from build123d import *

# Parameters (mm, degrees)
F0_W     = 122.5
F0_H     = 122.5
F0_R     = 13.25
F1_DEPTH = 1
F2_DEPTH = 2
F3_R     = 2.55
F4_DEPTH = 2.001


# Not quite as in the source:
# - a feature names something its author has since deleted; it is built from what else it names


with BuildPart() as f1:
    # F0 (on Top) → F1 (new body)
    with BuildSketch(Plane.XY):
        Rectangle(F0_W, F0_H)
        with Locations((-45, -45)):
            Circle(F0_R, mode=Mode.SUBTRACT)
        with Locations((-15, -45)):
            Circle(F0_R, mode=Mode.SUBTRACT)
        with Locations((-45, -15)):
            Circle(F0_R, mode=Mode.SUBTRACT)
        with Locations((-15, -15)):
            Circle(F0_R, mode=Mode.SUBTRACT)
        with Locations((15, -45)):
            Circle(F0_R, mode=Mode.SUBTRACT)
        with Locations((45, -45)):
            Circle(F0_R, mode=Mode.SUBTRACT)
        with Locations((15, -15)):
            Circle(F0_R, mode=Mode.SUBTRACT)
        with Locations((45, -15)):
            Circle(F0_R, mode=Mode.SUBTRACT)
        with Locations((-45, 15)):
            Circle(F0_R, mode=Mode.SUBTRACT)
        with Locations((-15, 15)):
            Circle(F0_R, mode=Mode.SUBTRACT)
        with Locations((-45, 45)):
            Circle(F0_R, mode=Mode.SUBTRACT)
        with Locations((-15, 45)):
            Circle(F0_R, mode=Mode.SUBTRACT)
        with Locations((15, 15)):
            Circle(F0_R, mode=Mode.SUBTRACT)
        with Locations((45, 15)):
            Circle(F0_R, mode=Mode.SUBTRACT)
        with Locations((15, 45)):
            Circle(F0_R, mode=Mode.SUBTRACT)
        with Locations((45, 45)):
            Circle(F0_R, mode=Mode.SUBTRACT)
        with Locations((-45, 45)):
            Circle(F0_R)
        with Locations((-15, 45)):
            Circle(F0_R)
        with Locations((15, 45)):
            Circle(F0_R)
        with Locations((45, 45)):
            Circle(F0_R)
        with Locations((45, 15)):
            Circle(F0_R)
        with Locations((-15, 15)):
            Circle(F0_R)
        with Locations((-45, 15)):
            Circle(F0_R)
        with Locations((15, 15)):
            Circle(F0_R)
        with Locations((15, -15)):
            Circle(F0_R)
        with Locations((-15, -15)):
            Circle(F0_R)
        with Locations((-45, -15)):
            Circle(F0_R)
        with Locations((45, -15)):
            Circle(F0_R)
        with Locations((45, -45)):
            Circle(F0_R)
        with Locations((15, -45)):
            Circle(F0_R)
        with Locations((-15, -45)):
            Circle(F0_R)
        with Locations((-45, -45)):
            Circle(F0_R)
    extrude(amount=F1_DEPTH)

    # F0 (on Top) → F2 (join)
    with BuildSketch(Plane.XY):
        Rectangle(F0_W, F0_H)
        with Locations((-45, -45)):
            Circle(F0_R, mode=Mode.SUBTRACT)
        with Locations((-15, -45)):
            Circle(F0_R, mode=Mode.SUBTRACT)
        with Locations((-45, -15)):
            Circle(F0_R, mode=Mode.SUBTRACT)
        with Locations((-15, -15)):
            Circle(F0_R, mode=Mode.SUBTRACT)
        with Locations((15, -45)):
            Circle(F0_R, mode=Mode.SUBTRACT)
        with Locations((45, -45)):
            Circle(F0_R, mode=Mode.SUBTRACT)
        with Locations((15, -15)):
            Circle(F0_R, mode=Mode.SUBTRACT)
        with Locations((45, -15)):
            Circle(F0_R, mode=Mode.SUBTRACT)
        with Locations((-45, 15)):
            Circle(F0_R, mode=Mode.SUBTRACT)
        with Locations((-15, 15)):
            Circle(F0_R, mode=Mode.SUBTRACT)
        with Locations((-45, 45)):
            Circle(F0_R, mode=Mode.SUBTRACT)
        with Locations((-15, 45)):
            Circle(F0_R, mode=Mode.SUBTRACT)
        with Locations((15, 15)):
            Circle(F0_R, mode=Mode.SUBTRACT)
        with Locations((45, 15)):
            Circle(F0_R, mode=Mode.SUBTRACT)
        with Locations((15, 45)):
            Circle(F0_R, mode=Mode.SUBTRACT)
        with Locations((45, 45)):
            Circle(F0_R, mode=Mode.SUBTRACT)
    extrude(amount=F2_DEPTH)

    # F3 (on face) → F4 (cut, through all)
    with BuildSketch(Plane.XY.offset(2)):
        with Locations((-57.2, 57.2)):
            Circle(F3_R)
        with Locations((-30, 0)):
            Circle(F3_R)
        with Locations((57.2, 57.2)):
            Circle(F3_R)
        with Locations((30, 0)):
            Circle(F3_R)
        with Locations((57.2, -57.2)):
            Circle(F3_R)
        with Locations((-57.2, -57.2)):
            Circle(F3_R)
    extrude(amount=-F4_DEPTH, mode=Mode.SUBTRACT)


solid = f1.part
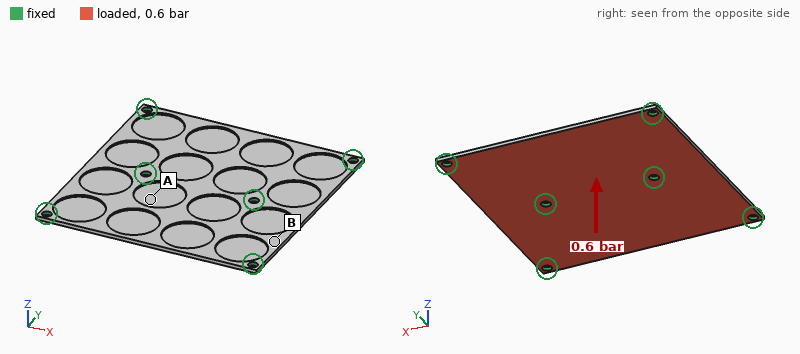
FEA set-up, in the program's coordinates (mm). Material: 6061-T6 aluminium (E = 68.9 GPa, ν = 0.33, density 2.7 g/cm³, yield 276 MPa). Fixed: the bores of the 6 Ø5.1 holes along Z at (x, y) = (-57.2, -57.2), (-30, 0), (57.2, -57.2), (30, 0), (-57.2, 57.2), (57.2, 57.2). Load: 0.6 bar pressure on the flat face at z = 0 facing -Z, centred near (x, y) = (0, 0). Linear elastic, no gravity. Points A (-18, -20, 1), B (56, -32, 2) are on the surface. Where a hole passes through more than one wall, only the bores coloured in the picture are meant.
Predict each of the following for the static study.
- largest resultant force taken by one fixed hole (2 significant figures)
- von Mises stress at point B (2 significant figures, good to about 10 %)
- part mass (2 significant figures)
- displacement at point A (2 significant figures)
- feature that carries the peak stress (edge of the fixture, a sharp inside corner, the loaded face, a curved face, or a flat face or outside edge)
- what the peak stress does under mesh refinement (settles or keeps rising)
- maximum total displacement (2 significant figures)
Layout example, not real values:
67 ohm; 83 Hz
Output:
260 N; 27 MPa; 57 g; 0.25 mm; edge of the fixture; keeps rising; 0.91 mm
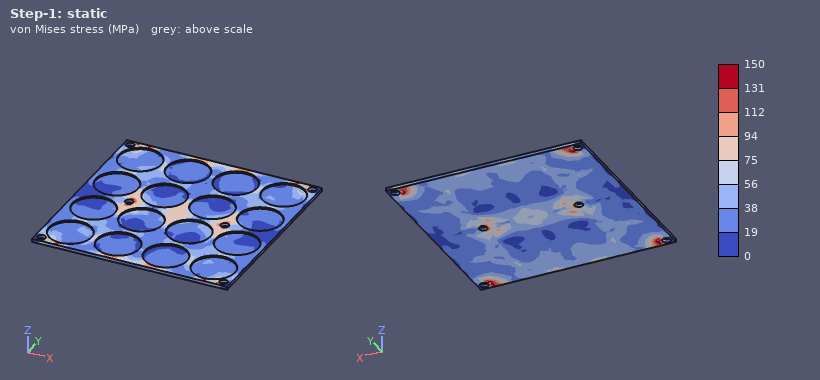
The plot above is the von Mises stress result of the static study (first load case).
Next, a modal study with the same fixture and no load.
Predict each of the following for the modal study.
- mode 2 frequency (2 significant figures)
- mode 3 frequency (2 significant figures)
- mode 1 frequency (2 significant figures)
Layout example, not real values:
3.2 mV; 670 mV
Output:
850 Hz; 1600 Hz; 810 Hz
